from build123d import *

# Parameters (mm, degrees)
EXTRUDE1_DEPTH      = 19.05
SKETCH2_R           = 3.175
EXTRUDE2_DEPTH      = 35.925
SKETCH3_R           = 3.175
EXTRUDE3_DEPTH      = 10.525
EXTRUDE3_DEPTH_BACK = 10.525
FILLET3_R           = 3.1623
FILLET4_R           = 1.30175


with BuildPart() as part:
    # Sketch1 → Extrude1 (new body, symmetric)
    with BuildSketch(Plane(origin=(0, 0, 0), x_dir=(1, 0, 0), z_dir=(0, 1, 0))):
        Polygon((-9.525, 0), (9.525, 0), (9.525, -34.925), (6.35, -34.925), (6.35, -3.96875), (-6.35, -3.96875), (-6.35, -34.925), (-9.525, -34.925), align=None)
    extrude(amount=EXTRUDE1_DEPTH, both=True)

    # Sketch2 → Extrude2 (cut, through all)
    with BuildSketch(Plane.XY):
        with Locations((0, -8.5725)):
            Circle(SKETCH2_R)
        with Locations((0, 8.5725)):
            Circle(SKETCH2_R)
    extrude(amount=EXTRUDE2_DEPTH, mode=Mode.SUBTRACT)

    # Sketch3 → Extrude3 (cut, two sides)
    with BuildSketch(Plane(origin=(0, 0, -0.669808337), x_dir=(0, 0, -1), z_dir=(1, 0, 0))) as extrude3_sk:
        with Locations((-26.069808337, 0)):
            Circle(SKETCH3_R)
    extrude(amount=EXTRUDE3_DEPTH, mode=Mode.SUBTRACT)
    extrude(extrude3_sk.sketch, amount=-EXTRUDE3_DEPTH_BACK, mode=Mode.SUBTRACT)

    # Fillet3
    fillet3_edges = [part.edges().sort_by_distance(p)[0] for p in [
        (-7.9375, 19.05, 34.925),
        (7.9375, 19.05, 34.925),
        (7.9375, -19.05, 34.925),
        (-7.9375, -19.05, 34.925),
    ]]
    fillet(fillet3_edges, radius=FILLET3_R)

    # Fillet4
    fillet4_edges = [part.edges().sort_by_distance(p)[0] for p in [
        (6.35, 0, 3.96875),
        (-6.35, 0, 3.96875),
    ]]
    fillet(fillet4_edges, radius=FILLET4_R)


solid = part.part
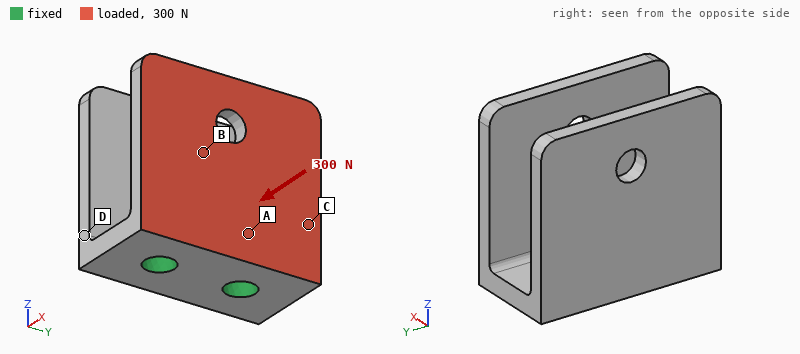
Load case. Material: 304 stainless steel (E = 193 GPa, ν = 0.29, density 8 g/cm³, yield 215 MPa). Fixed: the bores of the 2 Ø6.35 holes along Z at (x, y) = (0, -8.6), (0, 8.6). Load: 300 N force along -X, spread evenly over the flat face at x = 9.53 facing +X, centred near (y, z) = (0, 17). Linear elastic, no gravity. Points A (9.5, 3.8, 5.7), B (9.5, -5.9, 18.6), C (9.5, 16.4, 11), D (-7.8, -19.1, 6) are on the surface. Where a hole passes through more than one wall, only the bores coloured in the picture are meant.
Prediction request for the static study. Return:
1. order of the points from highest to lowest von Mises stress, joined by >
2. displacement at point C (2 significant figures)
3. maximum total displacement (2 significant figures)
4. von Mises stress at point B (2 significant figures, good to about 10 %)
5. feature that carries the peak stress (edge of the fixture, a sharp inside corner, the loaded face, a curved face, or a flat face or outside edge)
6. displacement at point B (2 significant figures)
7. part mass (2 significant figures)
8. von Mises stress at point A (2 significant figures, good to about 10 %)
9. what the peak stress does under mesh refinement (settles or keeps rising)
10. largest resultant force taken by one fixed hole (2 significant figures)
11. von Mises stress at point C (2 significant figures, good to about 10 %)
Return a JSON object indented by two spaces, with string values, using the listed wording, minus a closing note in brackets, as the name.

{
  "order of the points from highest to lowest von Mises stress, joined by >": "A > C > B > D",
  "displacement at point C": "12 µm",
  "maximum total displacement": "73 µm",
  "von Mises stress at point B": "16 MPa",
  "feature that carries the peak stress": "edge of the fixture",
  "displacement at point B": "28 µm",
  "part mass": "79 g",
  "von Mises stress at point A": "52 MPa",
  "what the peak stress does under mesh refinement": "keeps rising",
  "largest resultant force taken by one fixed hole": "150 N",
  "von Mises stress at point C": "37 MPa"
}
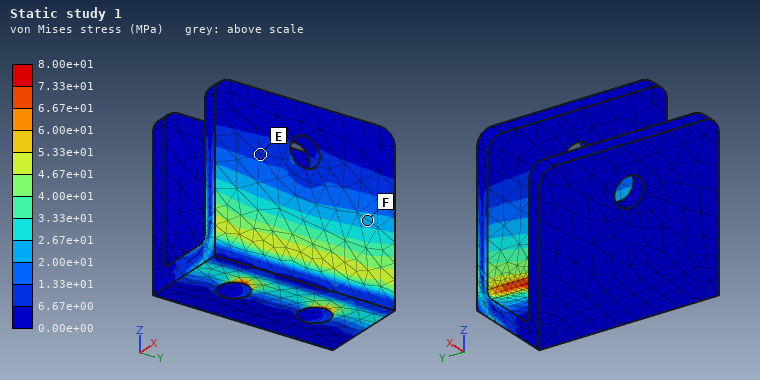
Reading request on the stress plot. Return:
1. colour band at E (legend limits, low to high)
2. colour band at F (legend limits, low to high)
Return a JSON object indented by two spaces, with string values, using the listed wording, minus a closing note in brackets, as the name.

{
  "colour band at E": "6.67e+00 to 1.33e+01 MPa",
  "colour band at F": "2.00e+01 to 2.67e+01 MPa"
}
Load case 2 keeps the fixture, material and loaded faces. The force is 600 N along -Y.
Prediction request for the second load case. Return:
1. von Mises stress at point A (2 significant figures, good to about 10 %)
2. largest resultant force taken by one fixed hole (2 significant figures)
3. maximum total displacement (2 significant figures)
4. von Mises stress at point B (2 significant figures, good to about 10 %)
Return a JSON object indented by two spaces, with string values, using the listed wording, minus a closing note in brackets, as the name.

{
  "von Mises stress at point A": "5.7 MPa",
  "largest resultant force taken by one fixed hole": "550 N",
  "maximum total displacement": "9.2 µm",
  "von Mises stress at point B": "8.4 MPa"
}
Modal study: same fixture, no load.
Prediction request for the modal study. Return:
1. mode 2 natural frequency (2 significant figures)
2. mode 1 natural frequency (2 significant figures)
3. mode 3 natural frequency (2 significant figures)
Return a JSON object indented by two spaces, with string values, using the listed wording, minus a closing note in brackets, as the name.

{
  "mode 2 natural frequency": "2200 Hz",
  "mode 1 natural frequency": "2200 Hz",
  "mode 3 natural frequency": "4700 Hz"
}
